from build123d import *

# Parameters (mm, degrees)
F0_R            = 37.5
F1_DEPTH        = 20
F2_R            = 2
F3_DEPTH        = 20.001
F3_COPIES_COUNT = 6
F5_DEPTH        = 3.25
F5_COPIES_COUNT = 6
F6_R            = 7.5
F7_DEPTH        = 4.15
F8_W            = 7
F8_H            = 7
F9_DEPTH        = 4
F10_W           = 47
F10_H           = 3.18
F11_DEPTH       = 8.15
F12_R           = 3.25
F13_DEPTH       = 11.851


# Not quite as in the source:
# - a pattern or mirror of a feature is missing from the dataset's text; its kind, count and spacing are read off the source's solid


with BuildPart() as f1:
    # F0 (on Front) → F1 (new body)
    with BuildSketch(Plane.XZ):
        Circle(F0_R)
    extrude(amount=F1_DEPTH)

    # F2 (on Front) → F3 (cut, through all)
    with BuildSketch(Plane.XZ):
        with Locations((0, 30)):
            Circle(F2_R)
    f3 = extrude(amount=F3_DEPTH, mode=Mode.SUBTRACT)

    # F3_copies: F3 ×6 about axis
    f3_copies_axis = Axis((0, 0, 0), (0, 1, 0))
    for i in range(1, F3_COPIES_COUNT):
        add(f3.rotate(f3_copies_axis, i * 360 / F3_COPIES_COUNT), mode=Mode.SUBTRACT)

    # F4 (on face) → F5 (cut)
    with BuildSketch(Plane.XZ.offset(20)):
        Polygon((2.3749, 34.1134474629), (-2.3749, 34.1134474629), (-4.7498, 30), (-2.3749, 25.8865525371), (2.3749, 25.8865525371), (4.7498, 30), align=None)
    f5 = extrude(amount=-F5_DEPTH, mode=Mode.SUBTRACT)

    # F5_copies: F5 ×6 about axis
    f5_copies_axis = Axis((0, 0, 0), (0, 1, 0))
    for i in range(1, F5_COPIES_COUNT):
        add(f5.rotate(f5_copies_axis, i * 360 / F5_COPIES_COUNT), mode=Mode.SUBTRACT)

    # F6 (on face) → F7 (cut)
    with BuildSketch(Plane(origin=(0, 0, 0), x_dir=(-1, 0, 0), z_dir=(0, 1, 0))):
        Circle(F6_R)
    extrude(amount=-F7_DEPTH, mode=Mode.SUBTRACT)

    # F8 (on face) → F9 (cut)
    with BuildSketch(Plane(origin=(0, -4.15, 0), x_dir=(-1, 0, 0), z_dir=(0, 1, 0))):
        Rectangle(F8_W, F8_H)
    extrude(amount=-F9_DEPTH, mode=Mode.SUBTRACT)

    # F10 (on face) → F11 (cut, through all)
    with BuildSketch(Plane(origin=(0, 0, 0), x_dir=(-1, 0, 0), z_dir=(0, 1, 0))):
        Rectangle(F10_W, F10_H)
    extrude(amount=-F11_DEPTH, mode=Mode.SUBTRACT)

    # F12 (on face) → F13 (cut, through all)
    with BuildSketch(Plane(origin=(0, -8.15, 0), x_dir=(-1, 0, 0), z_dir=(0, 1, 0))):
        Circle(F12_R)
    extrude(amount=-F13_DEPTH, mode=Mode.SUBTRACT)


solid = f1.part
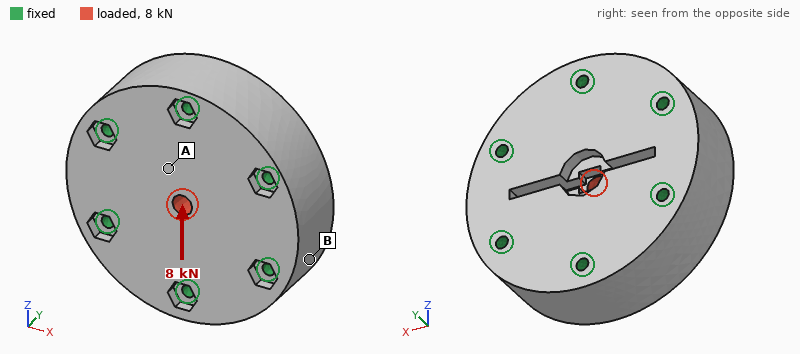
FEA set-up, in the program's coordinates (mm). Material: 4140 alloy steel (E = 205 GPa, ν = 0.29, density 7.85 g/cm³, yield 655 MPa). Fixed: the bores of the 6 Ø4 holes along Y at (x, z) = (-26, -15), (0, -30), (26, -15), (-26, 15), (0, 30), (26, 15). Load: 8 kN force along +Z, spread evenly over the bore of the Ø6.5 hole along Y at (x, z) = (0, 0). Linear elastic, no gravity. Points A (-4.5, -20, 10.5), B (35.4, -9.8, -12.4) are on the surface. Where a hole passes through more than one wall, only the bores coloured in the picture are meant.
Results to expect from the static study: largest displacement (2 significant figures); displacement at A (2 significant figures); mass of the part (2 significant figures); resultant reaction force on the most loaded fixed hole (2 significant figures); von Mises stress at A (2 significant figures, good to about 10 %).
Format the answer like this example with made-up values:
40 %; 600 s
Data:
2.0 µm; 1.0 µm; 660 g; 2.1 kN; 14 MPa
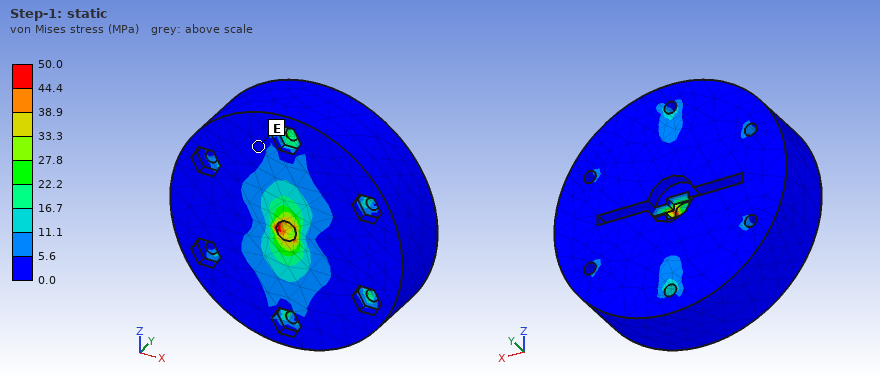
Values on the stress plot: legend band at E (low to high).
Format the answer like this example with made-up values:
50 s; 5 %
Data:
0.0 to 5.6 MPa
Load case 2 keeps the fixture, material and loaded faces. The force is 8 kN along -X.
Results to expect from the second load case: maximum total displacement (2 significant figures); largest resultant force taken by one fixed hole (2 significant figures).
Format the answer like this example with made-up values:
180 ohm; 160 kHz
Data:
2.0 µm; 1.8 kN
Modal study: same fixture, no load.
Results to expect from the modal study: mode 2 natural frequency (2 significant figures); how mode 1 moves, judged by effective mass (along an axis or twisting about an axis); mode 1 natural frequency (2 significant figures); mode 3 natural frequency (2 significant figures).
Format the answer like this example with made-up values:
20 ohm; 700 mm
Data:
34 kHz; along Y; 23 kHz; 35 kHz
